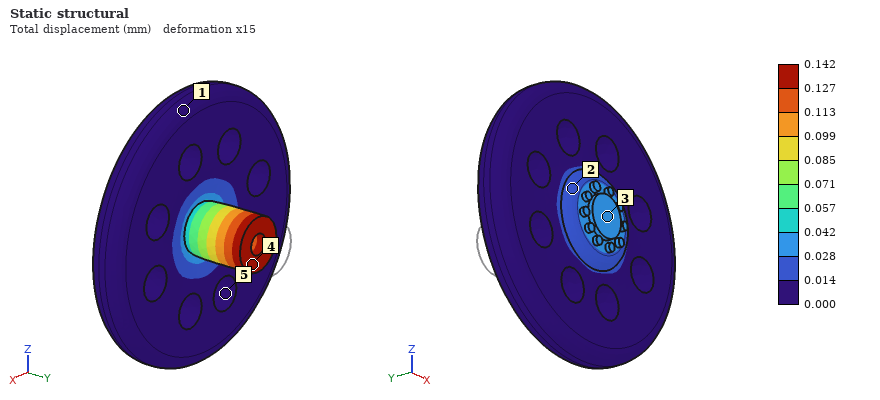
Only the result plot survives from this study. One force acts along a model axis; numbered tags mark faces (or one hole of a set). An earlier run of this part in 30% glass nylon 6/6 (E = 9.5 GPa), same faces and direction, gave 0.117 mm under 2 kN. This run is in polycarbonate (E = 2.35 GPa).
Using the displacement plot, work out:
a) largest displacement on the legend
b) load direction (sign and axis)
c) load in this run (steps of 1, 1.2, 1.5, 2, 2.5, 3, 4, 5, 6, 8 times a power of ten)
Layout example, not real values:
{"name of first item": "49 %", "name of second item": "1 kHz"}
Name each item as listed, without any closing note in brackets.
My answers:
{"largest displacement on the legend": "0.142 mm", "load direction": "-Y", "load in this run": "600 N"}
